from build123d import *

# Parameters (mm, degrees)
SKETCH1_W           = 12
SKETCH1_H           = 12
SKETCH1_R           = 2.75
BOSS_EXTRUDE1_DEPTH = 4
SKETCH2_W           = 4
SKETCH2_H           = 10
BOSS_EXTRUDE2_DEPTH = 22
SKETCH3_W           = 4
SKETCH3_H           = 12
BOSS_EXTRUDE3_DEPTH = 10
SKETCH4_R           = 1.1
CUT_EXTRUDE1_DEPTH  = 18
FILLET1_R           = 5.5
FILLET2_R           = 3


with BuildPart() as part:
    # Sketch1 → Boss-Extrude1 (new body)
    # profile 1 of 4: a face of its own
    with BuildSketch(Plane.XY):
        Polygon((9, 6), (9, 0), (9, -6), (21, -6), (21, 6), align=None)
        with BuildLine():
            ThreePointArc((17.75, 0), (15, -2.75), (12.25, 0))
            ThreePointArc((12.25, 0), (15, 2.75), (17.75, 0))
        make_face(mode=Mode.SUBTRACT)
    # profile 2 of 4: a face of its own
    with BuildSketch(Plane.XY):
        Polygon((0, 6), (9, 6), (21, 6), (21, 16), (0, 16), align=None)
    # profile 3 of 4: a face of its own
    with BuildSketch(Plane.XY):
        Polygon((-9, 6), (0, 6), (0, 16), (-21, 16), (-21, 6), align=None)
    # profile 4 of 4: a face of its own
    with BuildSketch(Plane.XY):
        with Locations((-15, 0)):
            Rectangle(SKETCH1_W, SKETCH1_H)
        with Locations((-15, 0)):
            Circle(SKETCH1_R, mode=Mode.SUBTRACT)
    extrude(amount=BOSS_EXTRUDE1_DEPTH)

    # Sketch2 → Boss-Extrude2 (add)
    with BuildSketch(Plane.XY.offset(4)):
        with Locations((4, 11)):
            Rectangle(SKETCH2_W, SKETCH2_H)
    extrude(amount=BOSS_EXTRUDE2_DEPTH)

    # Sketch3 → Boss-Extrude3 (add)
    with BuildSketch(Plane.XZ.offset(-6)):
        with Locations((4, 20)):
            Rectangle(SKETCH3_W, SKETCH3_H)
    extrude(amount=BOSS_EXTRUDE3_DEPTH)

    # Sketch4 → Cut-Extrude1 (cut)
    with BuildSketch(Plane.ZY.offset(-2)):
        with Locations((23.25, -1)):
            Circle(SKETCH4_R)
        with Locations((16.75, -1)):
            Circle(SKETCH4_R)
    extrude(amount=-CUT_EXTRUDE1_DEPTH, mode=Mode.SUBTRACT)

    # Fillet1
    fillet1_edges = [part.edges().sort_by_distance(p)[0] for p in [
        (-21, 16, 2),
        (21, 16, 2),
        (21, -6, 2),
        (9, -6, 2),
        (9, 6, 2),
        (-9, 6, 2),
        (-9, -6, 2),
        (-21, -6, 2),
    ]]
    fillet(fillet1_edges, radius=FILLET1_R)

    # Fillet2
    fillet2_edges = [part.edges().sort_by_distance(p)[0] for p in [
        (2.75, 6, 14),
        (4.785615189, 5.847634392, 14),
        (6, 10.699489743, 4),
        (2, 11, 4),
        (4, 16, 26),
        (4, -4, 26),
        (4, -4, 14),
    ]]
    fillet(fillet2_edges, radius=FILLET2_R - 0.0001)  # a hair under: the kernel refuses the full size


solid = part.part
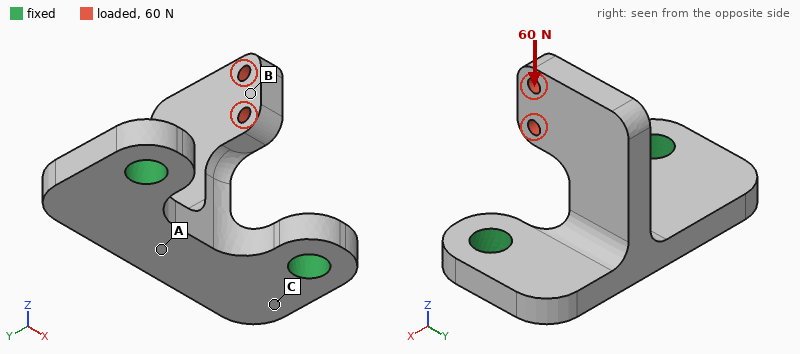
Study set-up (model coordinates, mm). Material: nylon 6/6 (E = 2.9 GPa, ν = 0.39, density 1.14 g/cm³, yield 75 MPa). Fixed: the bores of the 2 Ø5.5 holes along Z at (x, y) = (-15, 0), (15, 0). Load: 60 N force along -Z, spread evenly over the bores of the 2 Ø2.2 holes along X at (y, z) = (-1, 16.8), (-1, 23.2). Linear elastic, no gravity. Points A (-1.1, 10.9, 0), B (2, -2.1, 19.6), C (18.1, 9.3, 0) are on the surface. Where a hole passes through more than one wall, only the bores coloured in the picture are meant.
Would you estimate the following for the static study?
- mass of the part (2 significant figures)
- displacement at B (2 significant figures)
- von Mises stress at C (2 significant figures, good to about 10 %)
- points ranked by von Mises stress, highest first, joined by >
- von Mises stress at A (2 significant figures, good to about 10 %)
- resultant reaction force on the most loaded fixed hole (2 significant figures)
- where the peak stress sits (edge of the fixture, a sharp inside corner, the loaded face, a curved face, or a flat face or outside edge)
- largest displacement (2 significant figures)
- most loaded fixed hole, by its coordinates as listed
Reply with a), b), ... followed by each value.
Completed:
a) 4.4 g
b) 0.47 mm
c) 3.5 MPa
d) A > C > B
e) 6.4 MPa
f) 44 N
g) a curved face
h) 0.59 mm
i) (15, 0)
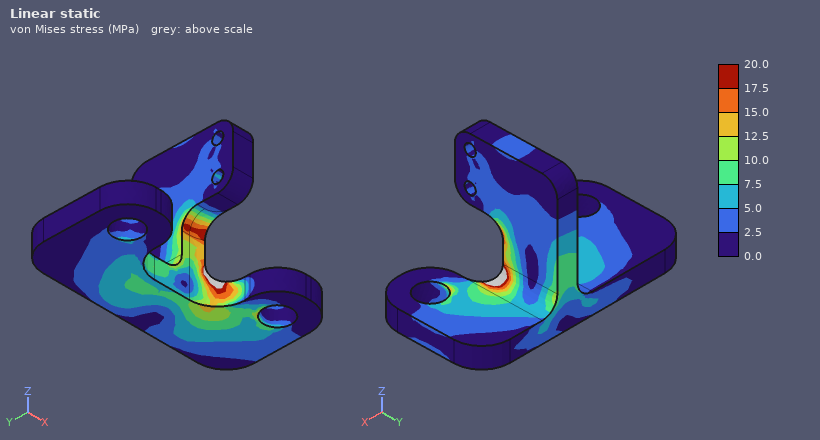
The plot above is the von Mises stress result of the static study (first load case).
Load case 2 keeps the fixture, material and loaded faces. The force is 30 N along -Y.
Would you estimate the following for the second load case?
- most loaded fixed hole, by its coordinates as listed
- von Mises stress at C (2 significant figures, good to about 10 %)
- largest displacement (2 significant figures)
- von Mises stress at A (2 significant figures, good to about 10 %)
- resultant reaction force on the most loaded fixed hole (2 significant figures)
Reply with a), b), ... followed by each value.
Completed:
a) (15, 0)
b) 5.1 MPa
c) 0.54 mm
d) 4.3 MPa
e) 27 N
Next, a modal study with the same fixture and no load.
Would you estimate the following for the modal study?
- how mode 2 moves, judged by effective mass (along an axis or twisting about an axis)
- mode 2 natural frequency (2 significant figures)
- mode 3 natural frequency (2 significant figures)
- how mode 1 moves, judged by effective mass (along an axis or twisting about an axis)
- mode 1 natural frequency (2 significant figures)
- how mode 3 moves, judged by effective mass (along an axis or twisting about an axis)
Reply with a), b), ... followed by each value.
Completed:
a) along X
b) 1300 Hz
c) 3200 Hz
d) along Y
e) 1200 Hz
f) along Z
